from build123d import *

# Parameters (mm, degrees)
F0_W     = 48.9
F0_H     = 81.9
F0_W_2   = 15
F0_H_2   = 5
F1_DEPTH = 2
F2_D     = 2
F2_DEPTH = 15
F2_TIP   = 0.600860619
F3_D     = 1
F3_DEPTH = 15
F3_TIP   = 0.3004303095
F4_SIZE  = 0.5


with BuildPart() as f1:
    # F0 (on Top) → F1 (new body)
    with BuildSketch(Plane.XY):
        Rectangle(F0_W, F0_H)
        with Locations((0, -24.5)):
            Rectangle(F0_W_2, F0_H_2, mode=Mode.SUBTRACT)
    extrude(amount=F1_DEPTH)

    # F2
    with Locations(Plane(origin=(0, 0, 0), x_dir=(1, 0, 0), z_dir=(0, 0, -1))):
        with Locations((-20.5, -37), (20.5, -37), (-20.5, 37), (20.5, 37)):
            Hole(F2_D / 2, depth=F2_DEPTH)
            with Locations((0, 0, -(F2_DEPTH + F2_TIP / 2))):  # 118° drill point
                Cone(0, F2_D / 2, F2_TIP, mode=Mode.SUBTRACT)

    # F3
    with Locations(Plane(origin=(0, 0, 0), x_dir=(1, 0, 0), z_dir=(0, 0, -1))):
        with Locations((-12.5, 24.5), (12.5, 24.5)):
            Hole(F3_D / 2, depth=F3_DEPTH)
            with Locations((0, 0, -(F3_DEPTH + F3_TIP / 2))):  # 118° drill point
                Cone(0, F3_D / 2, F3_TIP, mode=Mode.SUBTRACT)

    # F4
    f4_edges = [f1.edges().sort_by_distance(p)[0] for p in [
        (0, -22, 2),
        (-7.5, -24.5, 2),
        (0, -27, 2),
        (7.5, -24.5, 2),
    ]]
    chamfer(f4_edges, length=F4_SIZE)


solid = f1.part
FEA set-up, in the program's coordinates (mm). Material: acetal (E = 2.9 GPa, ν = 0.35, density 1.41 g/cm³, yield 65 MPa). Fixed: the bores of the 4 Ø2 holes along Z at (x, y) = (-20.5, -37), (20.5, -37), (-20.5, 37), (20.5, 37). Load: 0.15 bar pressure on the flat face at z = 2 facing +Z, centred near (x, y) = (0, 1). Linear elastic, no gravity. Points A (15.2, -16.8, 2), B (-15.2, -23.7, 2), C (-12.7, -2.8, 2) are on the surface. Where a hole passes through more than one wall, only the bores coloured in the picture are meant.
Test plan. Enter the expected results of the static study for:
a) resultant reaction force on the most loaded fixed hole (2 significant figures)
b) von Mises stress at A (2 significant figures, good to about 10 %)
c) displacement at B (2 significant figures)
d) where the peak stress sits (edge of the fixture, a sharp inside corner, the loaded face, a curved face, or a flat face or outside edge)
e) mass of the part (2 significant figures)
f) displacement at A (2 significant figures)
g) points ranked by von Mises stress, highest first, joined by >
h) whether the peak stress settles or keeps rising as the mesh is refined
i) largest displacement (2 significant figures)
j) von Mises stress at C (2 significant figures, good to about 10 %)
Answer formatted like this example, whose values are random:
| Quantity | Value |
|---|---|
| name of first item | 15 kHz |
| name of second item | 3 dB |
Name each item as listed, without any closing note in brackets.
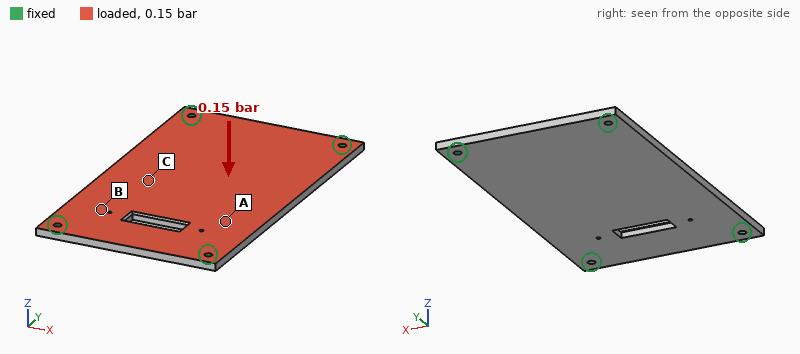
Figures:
| Quantity | Value |
|---|---|
| resultant reaction force on the most loaded fixed hole | 15 N |
| von Mises stress at A | 3.5 MPa |
| displacement at B | 0.37 mm |
| where the peak stress sits | edge of the fixture |
| mass of the part | 11 g |
| displacement at A | 0.59 mm |
| points ranked by von Mises stress, highest first, joined by > | C > A > B |
| whether the peak stress settles or keeps rising as the mesh is refined | keeps rising |
| largest displacement | 0.87 mm |
| von Mises stress at C | 5.6 MPa |
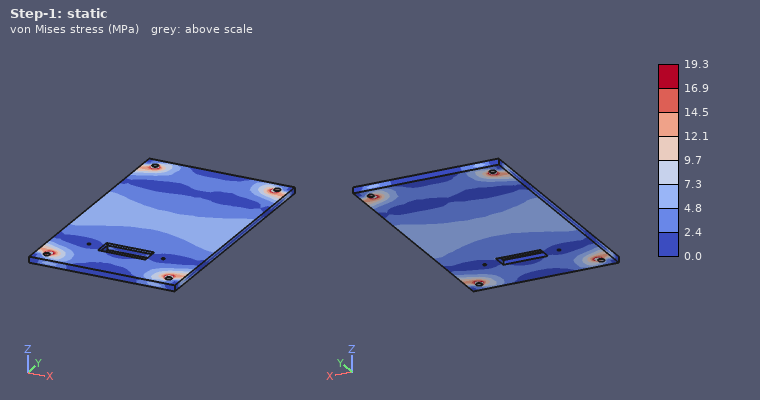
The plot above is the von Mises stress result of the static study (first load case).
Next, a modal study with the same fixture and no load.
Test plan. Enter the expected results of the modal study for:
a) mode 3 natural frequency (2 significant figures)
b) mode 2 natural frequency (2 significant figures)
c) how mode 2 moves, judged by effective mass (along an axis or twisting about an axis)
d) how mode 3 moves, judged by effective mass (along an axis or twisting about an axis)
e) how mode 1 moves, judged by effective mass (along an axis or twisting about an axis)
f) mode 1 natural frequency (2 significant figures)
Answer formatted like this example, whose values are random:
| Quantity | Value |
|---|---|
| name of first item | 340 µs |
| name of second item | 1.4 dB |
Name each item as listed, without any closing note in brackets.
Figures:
| Quantity | Value |
|---|---|
| mode 3 natural frequency | 1200 Hz |
| mode 2 natural frequency | 740 Hz |
| how mode 2 moves, judged by effective mass | twisting about Y |
| how mode 3 moves, judged by effective mass | twisting about X |
| how mode 1 moves, judged by effective mass | along Z |
| mode 1 natural frequency | 450 Hz |
